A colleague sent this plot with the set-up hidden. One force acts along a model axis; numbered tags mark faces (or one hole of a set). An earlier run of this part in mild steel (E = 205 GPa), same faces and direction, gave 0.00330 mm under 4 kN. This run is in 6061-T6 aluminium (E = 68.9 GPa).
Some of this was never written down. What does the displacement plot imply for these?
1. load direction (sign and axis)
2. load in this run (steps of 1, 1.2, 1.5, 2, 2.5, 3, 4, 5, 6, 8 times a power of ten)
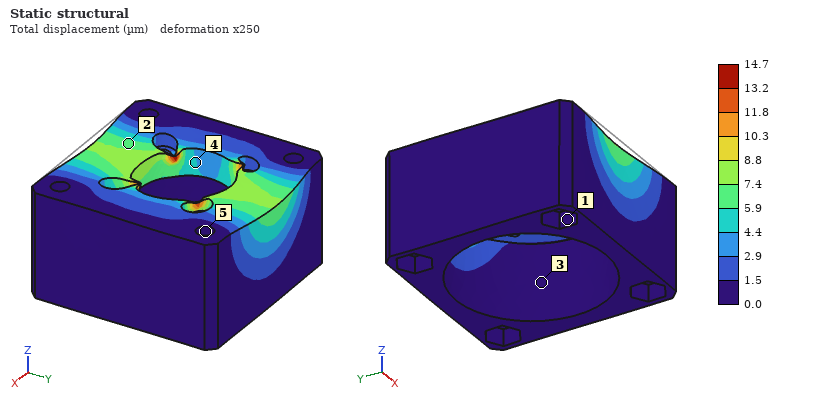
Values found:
+Y
6 kN
